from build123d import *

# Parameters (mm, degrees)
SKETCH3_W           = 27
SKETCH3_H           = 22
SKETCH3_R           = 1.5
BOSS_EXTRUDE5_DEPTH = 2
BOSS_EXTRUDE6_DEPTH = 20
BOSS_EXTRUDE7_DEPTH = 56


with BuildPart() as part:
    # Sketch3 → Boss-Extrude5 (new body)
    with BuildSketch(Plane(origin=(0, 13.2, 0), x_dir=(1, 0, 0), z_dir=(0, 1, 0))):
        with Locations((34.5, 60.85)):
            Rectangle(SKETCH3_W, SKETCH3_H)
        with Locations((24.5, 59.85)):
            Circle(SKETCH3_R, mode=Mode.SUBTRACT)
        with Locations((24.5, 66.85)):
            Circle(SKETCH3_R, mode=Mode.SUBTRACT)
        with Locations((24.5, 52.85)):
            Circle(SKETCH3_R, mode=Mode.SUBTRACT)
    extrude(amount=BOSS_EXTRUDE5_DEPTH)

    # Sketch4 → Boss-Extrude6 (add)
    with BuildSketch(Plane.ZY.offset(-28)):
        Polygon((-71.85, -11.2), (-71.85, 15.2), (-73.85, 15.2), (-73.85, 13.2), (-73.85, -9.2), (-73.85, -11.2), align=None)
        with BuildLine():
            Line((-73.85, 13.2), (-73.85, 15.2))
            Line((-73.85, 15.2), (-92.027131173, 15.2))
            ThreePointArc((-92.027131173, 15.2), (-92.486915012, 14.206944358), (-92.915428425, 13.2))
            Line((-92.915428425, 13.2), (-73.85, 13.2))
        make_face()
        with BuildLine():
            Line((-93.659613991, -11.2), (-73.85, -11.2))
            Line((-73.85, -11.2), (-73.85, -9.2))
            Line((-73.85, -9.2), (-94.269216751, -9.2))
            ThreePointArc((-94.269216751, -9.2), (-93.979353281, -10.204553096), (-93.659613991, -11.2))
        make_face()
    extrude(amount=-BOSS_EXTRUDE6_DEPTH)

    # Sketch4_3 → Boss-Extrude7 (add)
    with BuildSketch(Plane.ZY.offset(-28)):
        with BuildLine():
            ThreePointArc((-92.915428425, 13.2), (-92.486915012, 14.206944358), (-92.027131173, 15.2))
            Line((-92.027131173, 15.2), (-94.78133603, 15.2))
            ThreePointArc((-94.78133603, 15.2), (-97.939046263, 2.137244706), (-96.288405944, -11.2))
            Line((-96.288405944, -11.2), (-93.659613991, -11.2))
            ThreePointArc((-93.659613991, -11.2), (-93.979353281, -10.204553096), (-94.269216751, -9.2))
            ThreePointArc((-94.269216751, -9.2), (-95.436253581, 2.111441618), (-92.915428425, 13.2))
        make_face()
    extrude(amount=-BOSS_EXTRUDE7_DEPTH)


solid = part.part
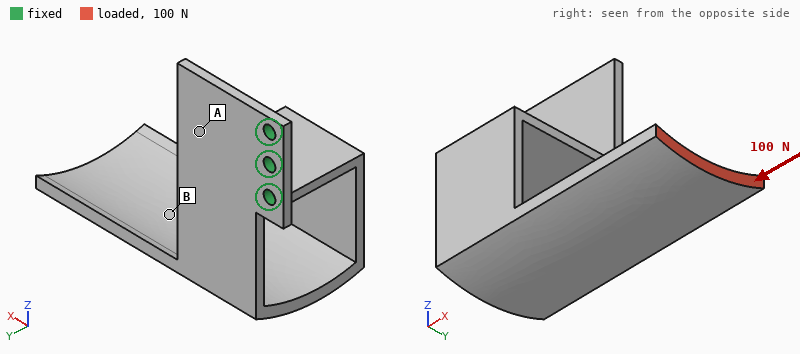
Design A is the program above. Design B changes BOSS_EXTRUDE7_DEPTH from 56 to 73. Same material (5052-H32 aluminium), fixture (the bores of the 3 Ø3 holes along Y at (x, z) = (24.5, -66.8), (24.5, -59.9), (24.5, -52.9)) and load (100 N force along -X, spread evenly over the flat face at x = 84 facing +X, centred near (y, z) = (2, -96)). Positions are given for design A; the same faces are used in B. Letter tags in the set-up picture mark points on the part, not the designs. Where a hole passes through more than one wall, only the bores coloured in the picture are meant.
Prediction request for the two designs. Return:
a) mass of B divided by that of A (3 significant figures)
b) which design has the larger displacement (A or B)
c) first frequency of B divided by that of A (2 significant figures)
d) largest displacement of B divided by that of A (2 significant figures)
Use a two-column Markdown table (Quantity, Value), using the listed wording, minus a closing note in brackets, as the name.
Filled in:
| Quantity | Value |
|---|---|
| mass of B divided by that of A | 1.15 |
| which design has the larger displacement | B |
| first frequency of B divided by that of A | 0.78 |
| largest displacement of B divided by that of A | 1.2 |
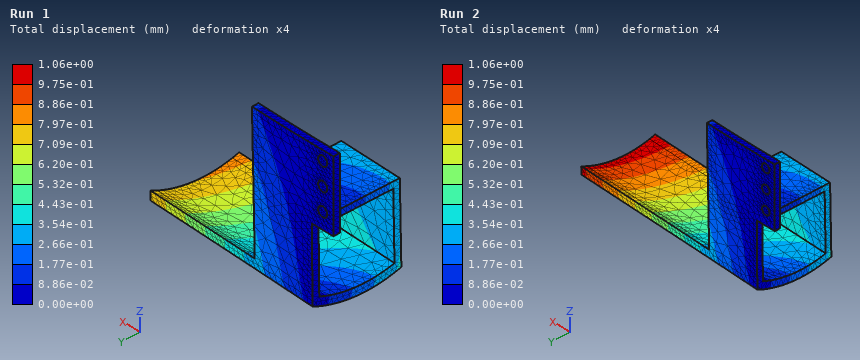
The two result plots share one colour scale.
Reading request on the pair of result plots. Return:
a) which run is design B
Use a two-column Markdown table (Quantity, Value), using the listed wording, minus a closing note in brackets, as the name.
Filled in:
| Quantity | Value |
|---|---|
| which run is design B | Run 2 |
